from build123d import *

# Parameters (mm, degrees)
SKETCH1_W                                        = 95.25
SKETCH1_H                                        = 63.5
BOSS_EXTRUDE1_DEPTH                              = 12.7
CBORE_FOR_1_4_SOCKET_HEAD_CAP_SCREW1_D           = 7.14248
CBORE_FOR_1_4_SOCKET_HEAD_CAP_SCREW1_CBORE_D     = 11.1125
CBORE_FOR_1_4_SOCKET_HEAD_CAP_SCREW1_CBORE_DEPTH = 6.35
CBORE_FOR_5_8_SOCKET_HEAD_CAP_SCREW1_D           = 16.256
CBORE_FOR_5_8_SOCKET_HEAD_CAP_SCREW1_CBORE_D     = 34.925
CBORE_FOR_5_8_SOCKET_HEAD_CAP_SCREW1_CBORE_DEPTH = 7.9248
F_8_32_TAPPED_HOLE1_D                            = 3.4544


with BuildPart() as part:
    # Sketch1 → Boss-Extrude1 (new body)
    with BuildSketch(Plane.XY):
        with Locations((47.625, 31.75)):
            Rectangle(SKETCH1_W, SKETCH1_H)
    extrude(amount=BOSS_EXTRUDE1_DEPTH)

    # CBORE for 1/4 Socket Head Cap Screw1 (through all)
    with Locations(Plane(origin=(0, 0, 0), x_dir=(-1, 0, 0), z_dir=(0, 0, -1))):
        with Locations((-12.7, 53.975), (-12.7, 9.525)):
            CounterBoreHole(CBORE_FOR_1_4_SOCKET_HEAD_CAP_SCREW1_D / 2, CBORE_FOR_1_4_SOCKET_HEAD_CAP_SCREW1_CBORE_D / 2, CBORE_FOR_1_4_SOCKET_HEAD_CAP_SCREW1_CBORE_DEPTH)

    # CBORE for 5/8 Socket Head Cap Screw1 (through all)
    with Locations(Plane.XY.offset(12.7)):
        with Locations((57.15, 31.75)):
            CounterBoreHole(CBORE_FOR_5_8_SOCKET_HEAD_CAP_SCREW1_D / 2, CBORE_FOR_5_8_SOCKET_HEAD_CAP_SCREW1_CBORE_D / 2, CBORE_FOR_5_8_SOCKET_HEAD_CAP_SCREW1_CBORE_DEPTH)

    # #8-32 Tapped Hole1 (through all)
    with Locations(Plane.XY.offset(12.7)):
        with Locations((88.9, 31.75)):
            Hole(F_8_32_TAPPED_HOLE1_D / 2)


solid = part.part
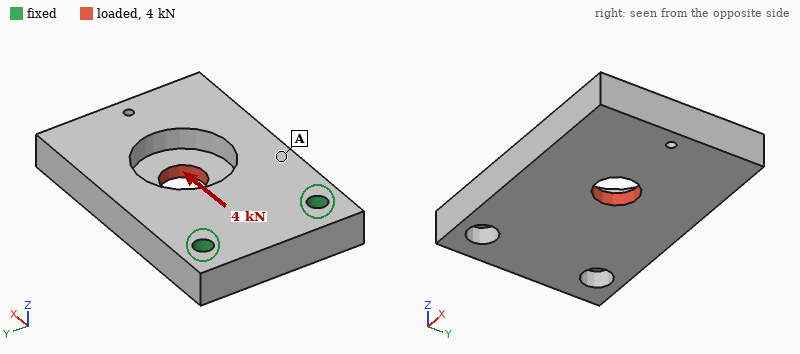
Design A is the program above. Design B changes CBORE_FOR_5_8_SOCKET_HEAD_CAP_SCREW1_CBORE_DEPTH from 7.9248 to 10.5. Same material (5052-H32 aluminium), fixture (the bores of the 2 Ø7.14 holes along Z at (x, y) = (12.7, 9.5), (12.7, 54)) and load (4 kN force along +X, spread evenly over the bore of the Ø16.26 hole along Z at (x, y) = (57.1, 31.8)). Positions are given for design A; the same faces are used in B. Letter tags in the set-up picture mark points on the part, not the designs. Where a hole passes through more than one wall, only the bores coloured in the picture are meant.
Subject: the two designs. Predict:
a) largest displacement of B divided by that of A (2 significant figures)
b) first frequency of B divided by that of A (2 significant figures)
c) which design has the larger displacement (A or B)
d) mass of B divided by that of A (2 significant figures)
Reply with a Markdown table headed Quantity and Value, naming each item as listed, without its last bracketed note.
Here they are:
| Quantity | Value |
|---|---|
| largest displacement of B divided by that of A | 1.3 |
| first frequency of B divided by that of A | 1.0 |
| which design has the larger displacement | B |
| mass of B divided by that of A | 0.97 |
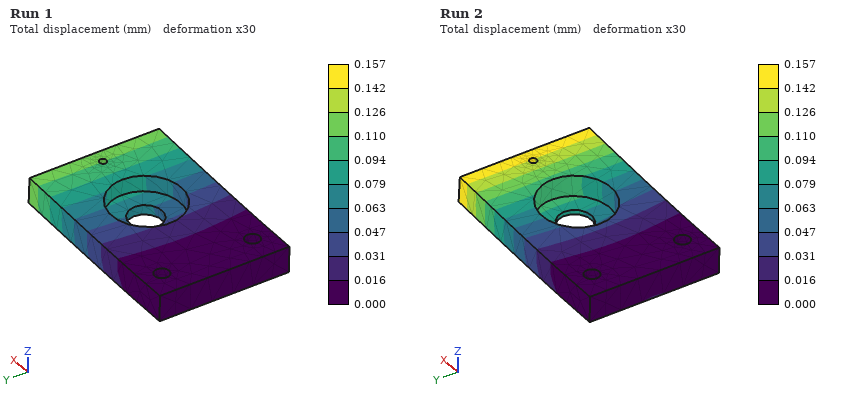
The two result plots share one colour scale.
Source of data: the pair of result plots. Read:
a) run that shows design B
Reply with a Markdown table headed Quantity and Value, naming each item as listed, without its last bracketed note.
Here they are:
| Quantity | Value |
|---|---|
| run that shows design B | Run 2 |
